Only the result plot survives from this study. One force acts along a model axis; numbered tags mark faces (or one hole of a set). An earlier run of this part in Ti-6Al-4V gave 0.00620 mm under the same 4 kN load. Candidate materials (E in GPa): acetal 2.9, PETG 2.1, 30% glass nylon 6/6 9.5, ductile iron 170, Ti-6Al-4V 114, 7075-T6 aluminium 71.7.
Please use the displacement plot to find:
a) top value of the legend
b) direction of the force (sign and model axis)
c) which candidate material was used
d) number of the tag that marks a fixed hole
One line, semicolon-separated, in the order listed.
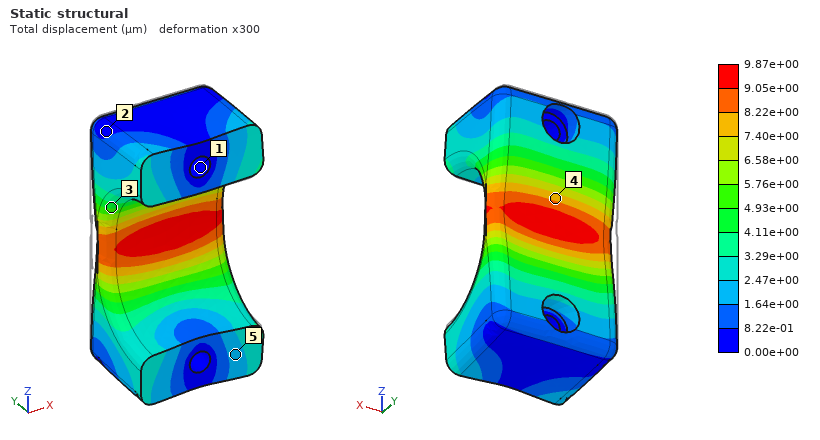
9.87e+00 µm; -Y; 7075-T6 aluminium; 1
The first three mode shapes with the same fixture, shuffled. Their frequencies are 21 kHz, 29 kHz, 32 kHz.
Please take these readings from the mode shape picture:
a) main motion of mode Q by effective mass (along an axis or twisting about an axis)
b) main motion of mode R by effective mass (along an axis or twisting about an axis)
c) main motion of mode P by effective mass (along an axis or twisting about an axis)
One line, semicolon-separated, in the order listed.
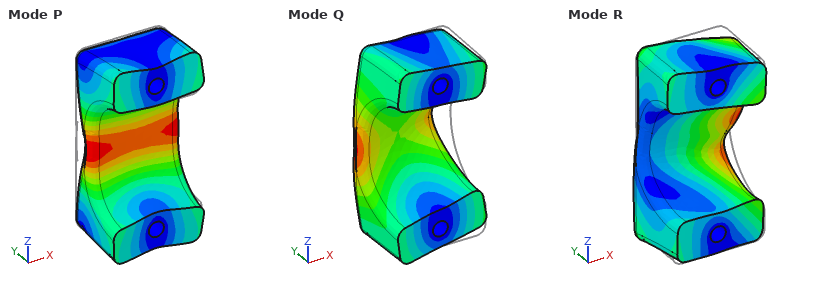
along X; along Z; along Y
